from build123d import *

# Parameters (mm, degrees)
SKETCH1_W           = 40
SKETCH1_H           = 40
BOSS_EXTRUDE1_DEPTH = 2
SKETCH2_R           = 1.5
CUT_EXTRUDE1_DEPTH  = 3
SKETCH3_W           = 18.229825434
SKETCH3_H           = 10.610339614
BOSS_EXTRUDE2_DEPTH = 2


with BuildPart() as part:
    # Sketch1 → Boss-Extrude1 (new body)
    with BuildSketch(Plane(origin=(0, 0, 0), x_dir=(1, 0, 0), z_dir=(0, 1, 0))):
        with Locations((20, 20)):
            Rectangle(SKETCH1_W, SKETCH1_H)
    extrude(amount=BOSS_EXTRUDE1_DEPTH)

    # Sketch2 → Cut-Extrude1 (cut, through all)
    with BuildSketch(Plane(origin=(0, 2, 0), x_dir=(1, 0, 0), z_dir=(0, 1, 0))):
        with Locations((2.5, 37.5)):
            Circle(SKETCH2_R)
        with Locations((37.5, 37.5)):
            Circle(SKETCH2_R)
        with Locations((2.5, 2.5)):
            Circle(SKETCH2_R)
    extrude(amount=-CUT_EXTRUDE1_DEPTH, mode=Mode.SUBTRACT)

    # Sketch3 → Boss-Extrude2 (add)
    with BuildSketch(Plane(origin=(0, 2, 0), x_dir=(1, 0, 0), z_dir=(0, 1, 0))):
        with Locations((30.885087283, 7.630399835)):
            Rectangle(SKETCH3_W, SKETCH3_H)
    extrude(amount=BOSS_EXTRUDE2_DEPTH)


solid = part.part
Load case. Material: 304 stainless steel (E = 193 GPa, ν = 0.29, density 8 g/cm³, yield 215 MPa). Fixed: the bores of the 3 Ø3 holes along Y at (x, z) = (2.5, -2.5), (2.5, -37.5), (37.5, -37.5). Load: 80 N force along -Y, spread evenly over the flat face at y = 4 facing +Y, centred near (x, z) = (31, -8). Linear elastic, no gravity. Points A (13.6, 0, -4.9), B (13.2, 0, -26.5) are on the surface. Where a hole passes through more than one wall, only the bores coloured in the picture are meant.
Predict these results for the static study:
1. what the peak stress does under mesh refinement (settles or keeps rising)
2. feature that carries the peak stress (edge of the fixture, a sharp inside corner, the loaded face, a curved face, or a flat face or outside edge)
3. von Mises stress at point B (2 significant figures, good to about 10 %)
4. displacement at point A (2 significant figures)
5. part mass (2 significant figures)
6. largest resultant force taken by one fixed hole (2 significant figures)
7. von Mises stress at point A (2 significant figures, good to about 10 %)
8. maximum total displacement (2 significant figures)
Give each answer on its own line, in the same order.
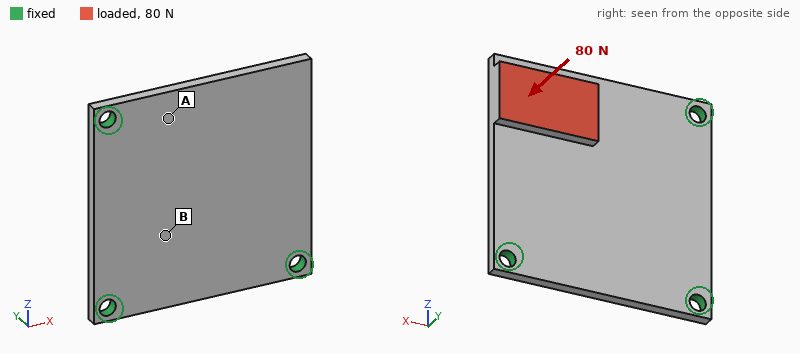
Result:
keeps rising
edge of the fixture
17 MPa
18 µm
28 g
54 N
40 MPa
96 µm
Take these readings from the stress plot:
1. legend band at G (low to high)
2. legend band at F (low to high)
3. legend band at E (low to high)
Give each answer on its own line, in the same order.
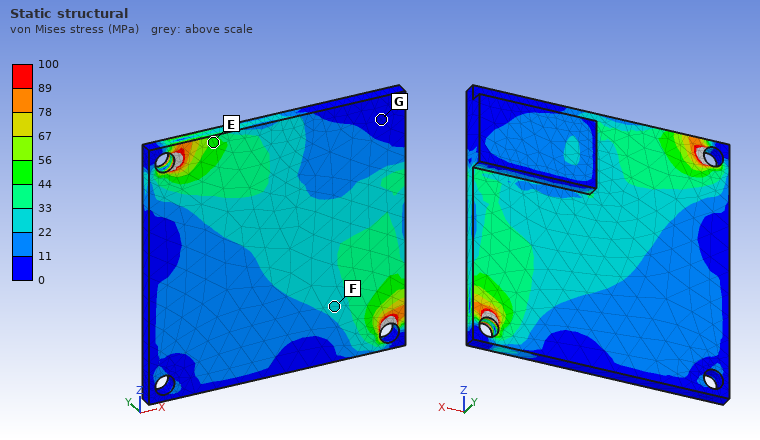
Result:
0 to 11 MPa
22 to 33 MPa
44 to 56 MPa
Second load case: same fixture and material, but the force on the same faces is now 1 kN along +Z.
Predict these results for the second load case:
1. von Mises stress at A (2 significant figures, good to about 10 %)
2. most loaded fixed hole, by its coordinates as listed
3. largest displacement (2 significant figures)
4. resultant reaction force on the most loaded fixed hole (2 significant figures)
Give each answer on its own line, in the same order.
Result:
98 MPa
(37.5, -37.5)
0.16 mm
560 N
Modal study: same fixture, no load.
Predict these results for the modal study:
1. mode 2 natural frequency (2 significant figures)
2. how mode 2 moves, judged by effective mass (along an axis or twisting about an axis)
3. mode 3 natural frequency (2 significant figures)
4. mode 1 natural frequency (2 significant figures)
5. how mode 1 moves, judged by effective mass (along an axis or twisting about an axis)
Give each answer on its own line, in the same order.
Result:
5800 Hz
along Y
7900 Hz
1900 Hz
along Y
